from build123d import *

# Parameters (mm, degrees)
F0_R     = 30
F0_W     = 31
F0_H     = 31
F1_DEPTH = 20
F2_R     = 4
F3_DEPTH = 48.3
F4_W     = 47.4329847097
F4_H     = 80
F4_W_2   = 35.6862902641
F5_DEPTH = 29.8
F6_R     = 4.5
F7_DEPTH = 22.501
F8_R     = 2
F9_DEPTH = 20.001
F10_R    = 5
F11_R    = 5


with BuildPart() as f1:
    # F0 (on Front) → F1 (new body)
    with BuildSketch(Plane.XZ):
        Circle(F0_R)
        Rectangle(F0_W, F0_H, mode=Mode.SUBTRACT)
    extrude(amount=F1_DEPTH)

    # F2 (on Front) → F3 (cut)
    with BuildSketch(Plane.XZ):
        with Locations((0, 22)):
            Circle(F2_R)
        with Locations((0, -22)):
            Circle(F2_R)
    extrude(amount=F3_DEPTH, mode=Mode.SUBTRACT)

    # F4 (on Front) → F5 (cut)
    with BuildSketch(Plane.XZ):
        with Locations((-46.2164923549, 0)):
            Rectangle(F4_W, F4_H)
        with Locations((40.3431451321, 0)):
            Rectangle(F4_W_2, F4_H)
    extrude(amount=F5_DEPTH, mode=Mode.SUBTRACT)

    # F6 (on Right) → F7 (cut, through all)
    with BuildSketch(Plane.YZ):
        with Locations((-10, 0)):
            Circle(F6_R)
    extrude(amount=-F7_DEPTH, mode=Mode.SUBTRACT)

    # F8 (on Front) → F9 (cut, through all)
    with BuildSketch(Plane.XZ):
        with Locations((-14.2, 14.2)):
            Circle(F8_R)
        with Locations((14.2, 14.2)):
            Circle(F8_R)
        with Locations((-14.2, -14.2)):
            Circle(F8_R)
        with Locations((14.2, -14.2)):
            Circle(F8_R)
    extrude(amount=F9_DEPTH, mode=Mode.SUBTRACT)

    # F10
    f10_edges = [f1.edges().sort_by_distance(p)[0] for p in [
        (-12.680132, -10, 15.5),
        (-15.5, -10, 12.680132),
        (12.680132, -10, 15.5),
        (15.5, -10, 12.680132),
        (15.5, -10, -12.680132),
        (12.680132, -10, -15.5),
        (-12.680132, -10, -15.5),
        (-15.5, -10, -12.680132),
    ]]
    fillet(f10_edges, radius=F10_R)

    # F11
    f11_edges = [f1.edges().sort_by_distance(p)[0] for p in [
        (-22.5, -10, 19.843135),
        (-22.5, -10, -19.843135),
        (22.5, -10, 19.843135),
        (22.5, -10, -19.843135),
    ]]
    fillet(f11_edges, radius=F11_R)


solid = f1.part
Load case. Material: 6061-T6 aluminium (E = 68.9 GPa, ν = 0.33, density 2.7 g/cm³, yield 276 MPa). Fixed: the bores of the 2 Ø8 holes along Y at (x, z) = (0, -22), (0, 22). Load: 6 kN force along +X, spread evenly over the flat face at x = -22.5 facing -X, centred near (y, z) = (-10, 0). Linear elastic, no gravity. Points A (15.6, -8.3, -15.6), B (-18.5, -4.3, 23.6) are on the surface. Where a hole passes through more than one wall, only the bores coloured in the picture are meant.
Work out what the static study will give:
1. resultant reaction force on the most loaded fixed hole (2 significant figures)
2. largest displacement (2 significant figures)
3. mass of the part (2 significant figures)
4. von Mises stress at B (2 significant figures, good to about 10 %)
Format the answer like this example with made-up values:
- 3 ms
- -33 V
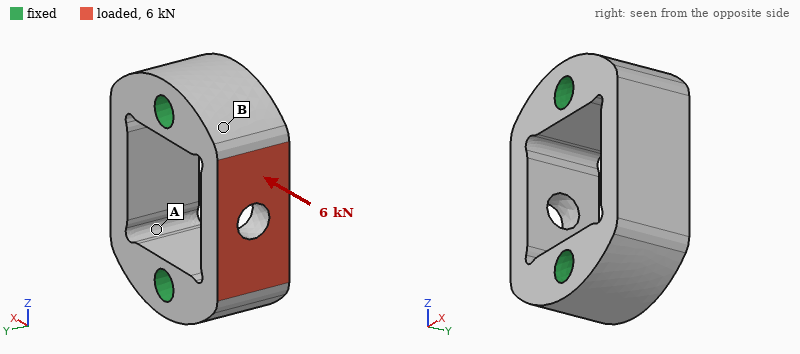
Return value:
- 3.5 kN
- 51 µm
- 71 g
- 34 MPa
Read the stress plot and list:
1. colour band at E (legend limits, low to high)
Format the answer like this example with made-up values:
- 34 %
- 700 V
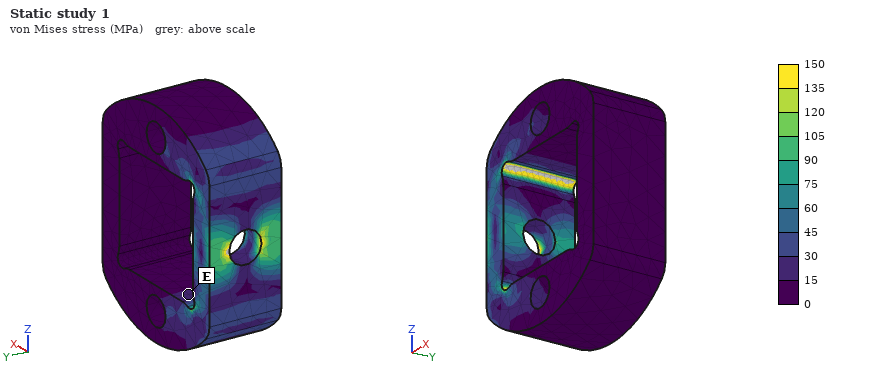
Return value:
- 15 to 30 MPa
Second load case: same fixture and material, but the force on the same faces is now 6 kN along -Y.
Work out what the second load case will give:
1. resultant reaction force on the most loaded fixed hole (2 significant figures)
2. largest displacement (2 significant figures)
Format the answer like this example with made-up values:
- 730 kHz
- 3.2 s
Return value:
- 3.0 kN
- 56 µm
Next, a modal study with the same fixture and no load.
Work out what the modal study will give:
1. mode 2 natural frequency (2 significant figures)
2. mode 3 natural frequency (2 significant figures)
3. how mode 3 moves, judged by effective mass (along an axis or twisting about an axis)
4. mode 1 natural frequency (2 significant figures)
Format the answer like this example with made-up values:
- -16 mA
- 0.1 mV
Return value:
- 17 kHz
- 18 kHz
- along Y
- 17 kHz
